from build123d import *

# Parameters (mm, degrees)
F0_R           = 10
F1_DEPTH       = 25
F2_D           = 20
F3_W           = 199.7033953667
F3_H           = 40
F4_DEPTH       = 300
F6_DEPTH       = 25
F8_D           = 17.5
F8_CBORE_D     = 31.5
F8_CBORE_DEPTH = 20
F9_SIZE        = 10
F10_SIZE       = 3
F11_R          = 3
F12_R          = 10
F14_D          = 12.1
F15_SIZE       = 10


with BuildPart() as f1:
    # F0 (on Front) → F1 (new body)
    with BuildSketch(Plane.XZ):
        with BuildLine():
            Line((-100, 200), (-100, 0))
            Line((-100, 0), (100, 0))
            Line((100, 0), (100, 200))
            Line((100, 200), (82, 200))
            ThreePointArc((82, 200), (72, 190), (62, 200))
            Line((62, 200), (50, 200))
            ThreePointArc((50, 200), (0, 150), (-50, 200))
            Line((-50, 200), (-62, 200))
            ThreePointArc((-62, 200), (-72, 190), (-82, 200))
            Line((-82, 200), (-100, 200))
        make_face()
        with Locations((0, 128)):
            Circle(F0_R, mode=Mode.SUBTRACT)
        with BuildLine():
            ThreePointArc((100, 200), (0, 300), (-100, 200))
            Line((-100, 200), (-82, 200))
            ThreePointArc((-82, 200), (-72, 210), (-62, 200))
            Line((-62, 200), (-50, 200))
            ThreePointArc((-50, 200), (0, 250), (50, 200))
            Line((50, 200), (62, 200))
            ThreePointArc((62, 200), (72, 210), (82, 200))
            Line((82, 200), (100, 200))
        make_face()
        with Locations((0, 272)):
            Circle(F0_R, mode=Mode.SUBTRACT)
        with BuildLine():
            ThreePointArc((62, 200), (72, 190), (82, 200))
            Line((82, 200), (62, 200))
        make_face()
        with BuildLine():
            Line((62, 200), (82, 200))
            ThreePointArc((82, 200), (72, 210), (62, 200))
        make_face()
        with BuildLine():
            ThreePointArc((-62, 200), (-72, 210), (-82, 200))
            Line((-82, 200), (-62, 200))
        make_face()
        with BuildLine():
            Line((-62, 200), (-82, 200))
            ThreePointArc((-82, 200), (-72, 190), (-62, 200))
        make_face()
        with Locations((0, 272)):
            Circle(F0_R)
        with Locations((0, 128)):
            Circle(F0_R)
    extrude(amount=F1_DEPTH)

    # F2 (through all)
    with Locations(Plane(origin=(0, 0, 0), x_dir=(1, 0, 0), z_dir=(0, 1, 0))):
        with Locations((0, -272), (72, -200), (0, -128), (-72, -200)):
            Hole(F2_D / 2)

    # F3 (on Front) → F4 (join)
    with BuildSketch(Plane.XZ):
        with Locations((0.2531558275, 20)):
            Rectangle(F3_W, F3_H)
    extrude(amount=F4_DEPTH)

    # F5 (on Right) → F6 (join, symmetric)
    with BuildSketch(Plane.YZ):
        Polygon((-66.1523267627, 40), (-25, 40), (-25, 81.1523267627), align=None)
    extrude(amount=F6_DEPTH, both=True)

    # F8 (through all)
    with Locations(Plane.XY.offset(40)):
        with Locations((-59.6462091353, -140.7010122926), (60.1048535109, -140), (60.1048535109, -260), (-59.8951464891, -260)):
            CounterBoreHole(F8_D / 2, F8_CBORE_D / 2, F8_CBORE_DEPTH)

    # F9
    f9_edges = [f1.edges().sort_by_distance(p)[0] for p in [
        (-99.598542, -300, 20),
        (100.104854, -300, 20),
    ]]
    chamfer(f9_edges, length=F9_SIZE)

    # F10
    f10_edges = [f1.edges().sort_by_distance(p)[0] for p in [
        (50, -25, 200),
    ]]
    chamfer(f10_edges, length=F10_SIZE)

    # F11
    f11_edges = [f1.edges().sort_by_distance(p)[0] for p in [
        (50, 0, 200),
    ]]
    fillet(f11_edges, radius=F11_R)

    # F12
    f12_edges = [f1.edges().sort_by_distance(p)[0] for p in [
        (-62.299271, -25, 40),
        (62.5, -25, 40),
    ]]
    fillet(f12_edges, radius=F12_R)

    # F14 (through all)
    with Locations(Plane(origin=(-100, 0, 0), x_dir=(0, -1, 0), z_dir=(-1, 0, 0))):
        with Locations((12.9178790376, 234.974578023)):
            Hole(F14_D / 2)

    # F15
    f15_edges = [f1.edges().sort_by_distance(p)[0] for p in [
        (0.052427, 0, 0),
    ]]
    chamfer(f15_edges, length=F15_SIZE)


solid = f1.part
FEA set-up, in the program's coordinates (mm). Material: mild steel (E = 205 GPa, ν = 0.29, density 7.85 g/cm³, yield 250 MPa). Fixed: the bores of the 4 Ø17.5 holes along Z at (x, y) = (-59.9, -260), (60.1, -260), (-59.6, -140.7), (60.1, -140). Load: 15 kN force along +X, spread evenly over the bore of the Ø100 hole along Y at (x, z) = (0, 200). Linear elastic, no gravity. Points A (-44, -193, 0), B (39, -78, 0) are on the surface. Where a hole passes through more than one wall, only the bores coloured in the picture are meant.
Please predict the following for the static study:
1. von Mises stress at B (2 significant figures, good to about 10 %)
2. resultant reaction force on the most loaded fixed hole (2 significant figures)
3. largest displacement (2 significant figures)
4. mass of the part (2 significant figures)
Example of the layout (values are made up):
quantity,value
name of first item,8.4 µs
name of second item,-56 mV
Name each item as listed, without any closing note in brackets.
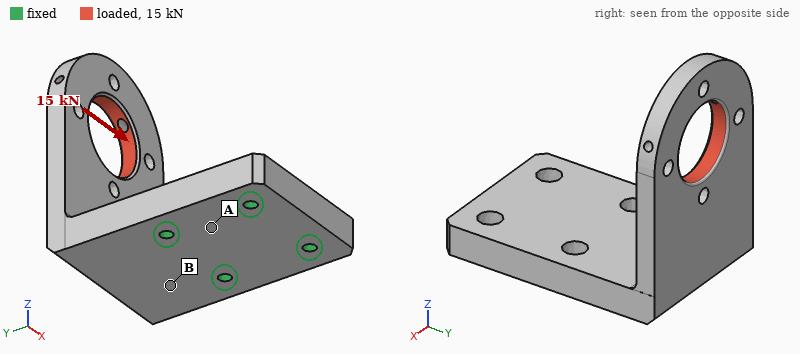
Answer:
quantity,value
von Mises stress at B,28 MPa
resultant reaction force on the most loaded fixed hole,30 kN
largest displacement,0.25 mm
mass of the part,26 kg
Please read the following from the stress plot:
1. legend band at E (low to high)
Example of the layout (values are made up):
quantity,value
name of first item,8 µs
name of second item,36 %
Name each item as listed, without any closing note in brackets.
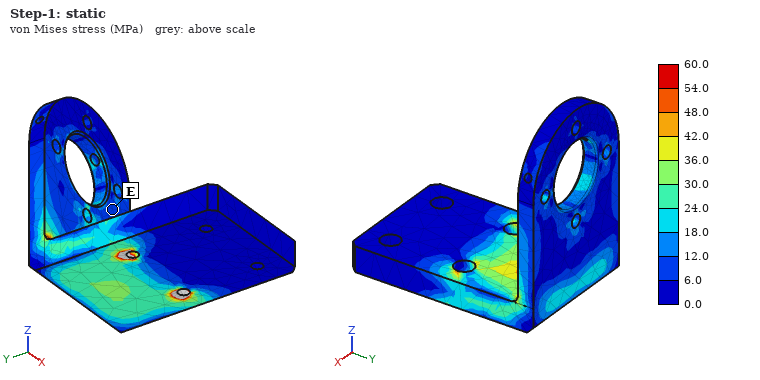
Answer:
quantity,value
legend band at E,6.0 to 12.0 MPa
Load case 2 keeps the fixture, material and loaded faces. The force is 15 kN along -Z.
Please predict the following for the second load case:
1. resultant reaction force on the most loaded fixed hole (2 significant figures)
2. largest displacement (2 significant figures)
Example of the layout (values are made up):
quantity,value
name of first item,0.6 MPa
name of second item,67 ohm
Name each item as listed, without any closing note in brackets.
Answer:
quantity,value
resultant reaction force on the most loaded fixed hole,16 kN
largest displacement,0.24 mm
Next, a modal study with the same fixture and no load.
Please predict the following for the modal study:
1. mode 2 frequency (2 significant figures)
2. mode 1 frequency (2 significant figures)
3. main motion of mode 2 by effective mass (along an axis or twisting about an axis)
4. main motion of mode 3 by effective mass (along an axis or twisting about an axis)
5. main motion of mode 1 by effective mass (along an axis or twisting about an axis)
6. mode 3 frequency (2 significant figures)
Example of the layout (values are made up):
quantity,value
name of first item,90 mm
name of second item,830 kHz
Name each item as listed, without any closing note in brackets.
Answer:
quantity,value
mode 2 frequency,620 Hz
mode 1 frequency,310 Hz
main motion of mode 2 by effective mass,along X
main motion of mode 3 by effective mass,along Z
main motion of mode 1 by effective mass,along Y
mode 3 frequency,770 Hz
